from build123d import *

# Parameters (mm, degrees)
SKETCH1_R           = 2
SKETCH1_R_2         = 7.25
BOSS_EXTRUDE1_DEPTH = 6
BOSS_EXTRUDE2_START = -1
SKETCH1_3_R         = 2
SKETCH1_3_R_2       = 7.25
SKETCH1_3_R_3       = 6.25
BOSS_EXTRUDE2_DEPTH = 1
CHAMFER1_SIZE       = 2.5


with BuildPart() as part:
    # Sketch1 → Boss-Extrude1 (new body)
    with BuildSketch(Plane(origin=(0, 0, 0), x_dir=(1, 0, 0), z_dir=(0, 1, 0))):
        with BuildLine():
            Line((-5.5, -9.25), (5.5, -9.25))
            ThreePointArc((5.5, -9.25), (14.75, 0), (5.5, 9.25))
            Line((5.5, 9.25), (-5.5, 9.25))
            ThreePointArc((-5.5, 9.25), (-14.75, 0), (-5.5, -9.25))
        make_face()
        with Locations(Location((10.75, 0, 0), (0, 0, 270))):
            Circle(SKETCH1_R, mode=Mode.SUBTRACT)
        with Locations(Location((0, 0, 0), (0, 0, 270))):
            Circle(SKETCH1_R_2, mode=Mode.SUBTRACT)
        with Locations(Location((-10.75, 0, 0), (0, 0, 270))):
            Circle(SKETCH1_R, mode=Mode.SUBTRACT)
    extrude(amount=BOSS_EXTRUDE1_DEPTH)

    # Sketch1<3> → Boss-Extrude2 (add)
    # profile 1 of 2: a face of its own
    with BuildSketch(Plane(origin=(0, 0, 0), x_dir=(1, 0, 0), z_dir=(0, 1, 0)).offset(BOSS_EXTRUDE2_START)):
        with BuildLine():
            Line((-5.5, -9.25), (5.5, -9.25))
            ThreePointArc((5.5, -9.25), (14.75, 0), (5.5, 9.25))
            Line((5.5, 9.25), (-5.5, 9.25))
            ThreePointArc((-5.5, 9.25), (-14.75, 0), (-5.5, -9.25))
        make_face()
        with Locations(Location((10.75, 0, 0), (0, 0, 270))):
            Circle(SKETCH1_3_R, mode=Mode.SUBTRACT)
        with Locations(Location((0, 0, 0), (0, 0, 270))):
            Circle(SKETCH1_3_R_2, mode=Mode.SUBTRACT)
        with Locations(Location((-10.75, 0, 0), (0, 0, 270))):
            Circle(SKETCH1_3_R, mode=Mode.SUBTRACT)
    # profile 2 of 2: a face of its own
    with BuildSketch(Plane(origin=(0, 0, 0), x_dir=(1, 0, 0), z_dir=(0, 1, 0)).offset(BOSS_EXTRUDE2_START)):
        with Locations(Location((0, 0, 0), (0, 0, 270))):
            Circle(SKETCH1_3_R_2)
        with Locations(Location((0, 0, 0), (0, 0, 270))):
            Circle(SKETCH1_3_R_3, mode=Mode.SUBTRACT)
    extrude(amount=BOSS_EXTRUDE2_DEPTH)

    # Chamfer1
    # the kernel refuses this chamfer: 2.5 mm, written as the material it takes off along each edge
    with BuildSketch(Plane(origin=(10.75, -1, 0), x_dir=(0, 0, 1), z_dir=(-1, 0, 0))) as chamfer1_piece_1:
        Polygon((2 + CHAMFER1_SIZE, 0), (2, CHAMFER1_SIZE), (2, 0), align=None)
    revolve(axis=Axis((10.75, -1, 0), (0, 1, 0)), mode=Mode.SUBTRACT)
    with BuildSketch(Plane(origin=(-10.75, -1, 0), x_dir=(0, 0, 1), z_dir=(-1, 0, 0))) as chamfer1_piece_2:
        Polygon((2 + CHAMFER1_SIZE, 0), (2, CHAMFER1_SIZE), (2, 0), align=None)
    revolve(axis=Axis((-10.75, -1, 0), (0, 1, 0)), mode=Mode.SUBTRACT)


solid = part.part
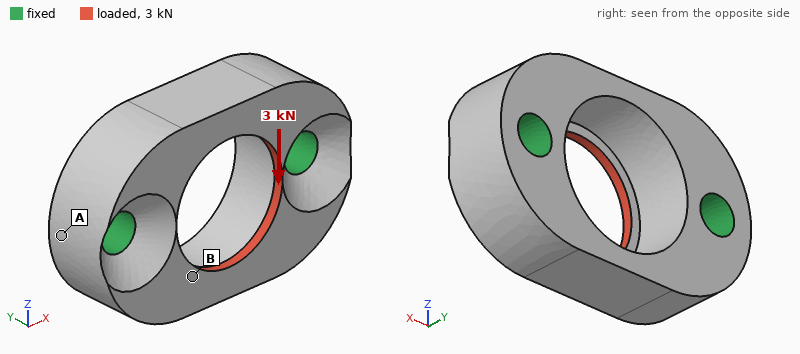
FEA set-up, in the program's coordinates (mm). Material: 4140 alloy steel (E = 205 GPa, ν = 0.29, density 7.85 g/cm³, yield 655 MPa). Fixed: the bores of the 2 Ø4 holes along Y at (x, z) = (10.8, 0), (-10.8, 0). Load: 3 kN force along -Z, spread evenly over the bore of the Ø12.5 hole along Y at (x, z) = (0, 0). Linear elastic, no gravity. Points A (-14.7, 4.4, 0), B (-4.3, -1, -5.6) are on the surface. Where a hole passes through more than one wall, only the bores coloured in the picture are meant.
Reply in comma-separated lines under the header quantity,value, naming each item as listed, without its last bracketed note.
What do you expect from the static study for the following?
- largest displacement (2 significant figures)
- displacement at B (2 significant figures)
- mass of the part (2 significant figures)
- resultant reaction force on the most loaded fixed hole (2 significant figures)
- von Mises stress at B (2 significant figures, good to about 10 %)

quantity,value
largest displacement,13 µm
displacement at B,7.6 µm
mass of the part,15 g
resultant reaction force on the most loaded fixed hole,1.5 kN
von Mises stress at B,110 MPa
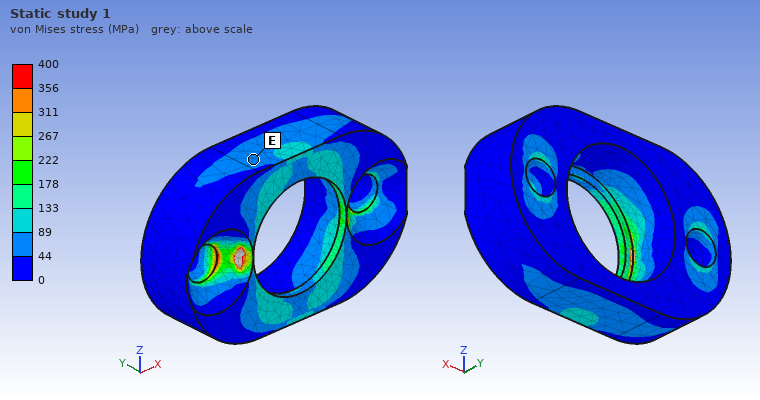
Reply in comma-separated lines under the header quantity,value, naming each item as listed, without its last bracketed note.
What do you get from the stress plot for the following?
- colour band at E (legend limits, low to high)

quantity,value
colour band at E,44 to 89 MPa
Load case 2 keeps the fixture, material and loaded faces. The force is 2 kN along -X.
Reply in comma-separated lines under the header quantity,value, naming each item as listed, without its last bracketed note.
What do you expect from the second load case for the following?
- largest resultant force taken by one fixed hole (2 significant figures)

quantity,value
largest resultant force taken by one fixed hole,1.0 kN
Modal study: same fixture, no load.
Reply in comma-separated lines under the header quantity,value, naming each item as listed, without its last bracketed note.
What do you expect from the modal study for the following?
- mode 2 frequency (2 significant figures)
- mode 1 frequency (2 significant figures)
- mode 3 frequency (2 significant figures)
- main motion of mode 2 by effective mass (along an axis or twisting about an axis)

quantity,value
mode 2 frequency,34 kHz
mode 1 frequency,31 kHz
mode 3 frequency,47 kHz
main motion of mode 2 by effective mass,along Y
